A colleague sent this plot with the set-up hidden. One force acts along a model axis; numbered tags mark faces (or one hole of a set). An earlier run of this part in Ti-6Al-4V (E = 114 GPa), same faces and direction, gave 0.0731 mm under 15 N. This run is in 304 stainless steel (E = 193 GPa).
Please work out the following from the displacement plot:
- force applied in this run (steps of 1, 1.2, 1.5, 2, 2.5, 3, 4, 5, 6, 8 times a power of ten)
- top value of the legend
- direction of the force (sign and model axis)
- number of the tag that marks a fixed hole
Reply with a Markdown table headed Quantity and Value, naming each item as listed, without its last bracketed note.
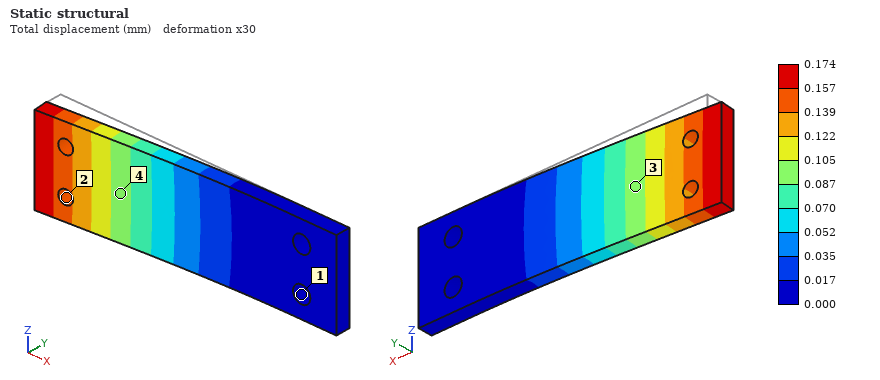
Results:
| Quantity | Value |
|---|---|
| force applied in this run | 60 N |
| top value of the legend | 0.174 mm |
| direction of the force | -Y |
| number of the tag that marks a fixed hole | 1 |
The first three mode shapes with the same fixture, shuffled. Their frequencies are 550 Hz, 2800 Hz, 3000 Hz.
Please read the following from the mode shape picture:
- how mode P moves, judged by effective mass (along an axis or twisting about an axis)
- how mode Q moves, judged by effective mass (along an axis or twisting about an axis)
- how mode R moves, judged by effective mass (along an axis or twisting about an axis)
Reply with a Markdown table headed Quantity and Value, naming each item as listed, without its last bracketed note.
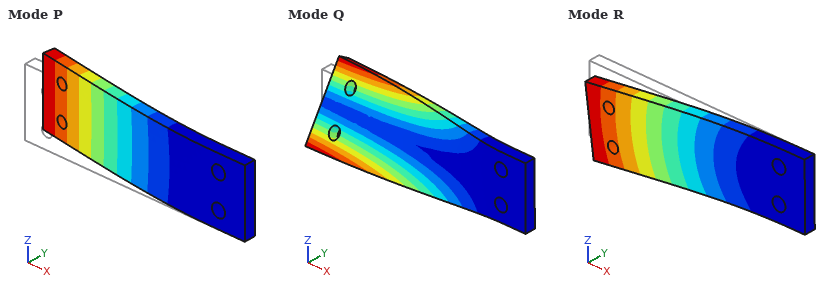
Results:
| Quantity | Value |
|---|---|
| how mode P moves, judged by effective mass | along Y |
| how mode Q moves, judged by effective mass | twisting about X |
| how mode R moves, judged by effective mass | along Z |
